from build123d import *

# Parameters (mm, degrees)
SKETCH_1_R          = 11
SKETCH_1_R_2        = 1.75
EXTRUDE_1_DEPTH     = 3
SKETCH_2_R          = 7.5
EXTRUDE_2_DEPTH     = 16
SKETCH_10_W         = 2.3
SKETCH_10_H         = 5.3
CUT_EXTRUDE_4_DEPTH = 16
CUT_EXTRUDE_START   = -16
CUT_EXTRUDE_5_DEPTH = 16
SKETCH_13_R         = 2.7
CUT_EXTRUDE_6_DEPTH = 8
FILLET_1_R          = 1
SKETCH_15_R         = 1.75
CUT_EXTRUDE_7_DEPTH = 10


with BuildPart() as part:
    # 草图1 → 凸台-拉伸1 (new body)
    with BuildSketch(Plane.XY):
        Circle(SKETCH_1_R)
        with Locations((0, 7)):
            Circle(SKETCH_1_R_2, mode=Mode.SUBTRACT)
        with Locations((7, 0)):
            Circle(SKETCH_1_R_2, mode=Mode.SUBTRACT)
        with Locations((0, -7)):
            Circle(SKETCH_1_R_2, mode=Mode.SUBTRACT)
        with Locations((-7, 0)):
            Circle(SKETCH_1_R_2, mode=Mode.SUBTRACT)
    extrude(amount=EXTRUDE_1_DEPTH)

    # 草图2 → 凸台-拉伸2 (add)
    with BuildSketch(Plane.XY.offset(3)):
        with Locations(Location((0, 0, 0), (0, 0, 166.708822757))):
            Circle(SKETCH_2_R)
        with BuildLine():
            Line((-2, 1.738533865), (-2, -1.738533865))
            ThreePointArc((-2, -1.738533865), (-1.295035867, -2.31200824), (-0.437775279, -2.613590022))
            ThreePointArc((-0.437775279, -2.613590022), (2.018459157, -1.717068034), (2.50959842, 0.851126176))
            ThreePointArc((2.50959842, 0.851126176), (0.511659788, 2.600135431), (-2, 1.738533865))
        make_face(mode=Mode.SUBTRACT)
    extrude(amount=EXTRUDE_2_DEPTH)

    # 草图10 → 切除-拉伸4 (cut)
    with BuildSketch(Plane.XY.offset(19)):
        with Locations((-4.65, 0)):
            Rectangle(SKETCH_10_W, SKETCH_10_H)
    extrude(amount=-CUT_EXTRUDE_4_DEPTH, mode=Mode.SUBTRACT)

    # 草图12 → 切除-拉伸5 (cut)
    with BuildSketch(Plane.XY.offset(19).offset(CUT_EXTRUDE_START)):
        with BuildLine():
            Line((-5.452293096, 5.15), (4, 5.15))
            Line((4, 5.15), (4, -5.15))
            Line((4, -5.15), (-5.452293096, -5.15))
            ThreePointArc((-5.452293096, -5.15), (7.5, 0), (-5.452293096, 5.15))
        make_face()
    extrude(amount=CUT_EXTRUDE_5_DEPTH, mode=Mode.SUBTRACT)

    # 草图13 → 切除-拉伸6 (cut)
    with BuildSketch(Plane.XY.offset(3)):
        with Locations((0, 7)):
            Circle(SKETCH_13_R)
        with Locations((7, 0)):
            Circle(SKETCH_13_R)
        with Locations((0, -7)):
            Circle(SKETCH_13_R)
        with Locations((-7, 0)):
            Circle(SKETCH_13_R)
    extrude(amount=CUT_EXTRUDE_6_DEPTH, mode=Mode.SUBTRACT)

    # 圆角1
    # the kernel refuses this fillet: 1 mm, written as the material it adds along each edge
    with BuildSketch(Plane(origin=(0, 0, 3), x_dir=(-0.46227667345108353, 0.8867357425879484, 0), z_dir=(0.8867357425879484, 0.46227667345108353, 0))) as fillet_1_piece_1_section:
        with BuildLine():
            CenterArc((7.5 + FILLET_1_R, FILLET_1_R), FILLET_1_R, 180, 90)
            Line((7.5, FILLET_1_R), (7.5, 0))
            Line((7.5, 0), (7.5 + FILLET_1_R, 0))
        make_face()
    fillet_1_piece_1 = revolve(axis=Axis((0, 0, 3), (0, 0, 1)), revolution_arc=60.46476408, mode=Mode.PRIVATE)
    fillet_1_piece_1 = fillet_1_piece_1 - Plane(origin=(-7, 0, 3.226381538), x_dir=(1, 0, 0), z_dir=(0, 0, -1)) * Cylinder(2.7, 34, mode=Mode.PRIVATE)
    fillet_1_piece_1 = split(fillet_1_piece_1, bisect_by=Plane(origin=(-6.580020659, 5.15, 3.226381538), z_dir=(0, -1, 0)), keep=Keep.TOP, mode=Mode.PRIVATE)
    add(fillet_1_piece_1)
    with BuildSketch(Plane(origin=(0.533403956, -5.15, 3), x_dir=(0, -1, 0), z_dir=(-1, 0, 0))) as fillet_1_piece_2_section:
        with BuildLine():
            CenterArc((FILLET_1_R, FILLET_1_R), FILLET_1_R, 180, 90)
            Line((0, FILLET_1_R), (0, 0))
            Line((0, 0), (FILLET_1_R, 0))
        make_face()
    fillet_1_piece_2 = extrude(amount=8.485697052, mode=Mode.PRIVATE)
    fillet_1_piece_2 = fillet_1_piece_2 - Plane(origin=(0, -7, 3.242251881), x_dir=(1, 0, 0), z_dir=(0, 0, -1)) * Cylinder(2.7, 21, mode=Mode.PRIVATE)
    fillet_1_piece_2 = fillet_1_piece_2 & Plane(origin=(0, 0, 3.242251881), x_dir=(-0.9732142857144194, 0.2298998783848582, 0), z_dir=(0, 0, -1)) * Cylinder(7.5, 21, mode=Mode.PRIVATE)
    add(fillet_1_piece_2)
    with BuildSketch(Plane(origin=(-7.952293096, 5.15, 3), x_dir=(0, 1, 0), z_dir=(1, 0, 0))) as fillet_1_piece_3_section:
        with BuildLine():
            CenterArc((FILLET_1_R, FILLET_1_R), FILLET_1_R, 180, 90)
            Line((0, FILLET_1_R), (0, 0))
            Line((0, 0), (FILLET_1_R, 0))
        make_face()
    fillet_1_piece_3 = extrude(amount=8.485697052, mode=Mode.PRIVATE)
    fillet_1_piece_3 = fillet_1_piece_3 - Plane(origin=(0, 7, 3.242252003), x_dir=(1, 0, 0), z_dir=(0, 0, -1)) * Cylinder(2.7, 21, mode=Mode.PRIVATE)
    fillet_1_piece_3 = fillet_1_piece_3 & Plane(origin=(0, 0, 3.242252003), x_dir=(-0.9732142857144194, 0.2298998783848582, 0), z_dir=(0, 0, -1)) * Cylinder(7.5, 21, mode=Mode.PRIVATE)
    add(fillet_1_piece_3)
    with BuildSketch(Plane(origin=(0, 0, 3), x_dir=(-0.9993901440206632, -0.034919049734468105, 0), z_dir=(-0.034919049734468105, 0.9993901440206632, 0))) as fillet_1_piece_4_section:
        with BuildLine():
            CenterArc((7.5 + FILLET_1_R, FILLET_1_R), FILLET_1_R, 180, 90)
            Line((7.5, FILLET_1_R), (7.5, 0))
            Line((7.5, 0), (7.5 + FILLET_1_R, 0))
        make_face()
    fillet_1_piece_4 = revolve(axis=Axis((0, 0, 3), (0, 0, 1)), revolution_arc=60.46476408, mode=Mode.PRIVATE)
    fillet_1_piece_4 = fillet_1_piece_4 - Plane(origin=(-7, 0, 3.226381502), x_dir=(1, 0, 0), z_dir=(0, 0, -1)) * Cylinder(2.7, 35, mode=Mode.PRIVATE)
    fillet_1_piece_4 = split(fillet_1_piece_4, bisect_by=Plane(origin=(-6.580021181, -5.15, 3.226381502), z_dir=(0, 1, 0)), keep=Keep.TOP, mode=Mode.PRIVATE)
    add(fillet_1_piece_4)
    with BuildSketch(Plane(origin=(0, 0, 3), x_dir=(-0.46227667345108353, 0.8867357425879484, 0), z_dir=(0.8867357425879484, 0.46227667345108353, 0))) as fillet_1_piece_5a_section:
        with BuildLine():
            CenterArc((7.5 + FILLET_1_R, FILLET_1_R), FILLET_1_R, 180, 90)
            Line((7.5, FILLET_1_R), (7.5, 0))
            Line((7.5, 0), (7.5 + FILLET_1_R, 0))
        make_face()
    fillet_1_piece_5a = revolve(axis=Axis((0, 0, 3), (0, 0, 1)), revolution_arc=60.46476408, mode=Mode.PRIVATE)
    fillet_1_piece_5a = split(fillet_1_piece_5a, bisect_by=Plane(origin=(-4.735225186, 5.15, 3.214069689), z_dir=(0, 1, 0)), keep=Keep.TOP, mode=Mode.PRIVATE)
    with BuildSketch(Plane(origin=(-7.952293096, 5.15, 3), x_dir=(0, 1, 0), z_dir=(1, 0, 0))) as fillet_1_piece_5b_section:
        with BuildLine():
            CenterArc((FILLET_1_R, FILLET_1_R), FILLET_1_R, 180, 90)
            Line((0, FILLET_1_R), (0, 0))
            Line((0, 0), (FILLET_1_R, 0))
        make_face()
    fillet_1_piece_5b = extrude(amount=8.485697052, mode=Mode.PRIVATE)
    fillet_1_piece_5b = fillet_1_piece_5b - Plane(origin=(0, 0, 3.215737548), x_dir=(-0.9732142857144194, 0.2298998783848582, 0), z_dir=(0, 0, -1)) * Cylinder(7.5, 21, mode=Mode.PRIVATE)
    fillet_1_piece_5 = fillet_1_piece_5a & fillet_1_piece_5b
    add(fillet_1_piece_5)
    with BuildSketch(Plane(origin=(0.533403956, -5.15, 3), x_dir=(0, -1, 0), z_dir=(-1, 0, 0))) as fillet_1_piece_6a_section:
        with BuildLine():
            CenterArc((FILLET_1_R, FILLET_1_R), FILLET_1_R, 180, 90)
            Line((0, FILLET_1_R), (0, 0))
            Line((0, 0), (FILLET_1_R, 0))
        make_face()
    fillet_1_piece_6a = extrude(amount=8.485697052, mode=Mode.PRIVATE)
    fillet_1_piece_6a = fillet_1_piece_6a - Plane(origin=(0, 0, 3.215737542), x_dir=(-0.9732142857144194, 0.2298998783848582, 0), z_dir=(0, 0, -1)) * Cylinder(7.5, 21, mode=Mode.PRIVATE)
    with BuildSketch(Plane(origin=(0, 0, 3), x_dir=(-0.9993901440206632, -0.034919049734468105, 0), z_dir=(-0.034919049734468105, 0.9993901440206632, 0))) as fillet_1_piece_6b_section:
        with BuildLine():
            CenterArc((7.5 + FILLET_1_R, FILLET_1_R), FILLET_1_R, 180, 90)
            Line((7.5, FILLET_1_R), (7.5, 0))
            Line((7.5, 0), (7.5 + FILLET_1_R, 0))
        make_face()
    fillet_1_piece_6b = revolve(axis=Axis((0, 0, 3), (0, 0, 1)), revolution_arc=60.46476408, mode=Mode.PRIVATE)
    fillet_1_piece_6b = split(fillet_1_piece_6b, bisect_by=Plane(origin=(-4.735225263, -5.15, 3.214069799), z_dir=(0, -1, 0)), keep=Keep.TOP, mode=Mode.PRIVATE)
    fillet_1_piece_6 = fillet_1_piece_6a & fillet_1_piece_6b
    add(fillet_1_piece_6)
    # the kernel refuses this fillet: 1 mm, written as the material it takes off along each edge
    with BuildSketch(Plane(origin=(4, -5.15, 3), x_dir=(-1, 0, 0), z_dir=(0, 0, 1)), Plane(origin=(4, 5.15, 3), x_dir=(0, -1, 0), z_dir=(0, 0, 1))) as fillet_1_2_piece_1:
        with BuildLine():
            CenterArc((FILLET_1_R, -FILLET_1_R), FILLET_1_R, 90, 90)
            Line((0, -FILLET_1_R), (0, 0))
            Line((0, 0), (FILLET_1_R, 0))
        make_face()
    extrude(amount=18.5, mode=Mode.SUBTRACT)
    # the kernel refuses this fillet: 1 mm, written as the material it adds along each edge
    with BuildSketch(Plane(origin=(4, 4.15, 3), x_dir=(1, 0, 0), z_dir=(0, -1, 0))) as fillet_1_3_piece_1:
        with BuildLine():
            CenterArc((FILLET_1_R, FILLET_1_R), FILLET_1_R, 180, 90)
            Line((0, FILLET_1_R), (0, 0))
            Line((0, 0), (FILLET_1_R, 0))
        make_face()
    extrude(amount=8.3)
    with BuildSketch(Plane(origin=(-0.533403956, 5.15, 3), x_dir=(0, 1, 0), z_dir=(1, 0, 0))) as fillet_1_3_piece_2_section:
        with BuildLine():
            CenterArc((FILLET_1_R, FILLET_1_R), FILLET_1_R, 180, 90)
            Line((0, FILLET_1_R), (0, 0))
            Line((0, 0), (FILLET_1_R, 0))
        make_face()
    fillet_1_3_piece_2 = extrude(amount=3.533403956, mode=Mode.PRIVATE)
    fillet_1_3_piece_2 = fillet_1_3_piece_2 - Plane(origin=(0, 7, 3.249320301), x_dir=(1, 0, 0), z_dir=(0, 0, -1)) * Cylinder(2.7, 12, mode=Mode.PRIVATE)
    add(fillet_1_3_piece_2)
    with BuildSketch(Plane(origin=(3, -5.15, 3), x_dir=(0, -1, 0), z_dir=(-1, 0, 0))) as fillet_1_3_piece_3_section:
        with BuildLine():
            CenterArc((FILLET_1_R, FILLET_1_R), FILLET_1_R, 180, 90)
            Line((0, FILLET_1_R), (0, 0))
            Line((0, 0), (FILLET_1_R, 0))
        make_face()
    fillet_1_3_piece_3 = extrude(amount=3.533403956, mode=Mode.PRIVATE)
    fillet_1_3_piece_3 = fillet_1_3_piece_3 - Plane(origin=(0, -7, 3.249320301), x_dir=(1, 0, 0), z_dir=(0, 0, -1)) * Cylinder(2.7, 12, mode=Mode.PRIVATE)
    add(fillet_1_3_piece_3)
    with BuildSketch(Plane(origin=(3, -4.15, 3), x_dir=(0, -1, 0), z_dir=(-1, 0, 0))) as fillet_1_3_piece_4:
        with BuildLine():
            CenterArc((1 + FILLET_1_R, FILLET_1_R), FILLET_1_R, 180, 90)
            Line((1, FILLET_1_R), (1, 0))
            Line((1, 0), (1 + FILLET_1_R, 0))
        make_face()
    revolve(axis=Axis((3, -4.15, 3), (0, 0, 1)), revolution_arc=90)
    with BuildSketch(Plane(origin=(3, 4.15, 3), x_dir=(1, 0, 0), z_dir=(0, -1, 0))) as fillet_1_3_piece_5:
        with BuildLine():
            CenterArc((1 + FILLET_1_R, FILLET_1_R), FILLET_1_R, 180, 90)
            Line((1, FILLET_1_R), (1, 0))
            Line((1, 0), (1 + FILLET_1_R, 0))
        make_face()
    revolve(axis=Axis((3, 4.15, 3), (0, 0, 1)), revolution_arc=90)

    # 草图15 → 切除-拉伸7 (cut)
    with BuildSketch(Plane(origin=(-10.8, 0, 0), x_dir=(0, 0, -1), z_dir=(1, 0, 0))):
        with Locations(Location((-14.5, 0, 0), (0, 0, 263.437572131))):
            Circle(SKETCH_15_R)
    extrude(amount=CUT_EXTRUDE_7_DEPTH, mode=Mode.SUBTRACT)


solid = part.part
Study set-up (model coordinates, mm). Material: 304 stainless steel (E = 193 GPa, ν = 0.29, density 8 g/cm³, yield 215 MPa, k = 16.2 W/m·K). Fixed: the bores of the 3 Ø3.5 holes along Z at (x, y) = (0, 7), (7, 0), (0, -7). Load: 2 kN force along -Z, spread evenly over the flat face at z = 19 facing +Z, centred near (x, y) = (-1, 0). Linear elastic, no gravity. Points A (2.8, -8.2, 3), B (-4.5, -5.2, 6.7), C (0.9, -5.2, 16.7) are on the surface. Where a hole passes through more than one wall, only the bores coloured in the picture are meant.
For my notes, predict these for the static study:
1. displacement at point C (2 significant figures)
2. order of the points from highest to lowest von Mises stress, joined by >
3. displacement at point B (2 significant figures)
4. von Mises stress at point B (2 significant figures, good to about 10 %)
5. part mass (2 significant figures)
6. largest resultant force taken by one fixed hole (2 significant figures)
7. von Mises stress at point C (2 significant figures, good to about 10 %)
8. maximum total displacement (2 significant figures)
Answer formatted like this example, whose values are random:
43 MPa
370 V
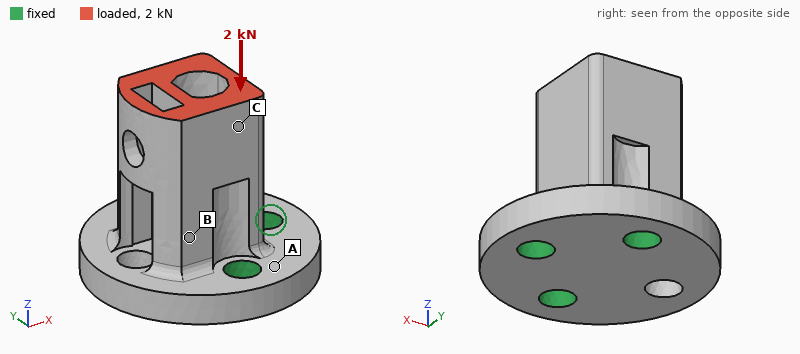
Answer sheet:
7.5 µm
B > C > A
5.0 µm
46 MPa
17 g
960 N
24 MPa
12 µm
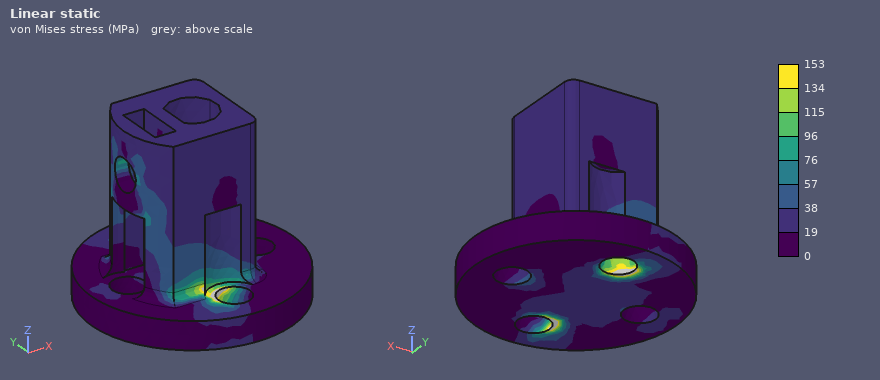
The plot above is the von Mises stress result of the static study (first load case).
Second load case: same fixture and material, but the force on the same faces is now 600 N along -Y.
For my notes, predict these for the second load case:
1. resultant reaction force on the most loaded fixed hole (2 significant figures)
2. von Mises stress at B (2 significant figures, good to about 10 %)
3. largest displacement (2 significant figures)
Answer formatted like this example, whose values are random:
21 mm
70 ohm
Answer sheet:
890 N
55 MPa
16 µm
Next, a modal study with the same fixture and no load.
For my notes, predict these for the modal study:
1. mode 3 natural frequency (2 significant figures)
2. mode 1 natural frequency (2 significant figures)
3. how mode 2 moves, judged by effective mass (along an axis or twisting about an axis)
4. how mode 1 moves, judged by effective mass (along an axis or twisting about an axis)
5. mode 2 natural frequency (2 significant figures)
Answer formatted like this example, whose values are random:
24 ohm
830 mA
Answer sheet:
32 kHz
14 kHz
along Y
along X
18 kHz
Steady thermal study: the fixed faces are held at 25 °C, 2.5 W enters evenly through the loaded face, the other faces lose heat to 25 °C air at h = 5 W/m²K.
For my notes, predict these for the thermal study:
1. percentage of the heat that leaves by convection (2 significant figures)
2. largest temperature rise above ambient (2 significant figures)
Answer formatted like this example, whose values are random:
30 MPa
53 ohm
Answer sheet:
5.6 %
43 K
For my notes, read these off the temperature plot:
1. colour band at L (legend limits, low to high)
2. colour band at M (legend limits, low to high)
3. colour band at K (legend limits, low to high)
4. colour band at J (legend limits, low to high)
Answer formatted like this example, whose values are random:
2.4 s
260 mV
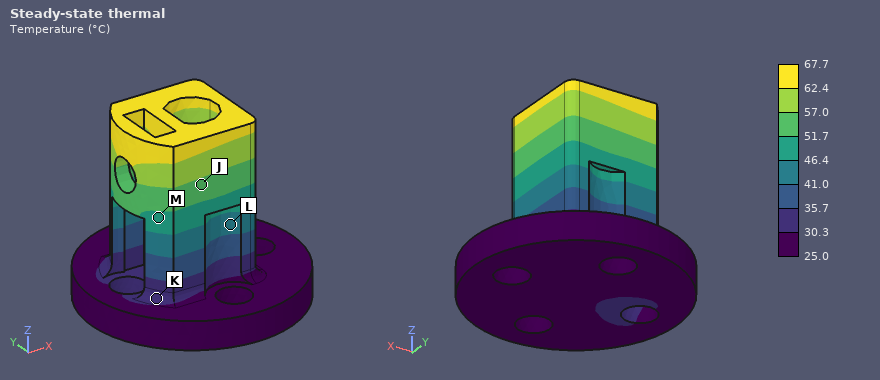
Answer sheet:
41.0 to 46.4 °C
46.4 to 51.7 °C
30.3 to 35.7 °C
51.7 to 57.0 °C
